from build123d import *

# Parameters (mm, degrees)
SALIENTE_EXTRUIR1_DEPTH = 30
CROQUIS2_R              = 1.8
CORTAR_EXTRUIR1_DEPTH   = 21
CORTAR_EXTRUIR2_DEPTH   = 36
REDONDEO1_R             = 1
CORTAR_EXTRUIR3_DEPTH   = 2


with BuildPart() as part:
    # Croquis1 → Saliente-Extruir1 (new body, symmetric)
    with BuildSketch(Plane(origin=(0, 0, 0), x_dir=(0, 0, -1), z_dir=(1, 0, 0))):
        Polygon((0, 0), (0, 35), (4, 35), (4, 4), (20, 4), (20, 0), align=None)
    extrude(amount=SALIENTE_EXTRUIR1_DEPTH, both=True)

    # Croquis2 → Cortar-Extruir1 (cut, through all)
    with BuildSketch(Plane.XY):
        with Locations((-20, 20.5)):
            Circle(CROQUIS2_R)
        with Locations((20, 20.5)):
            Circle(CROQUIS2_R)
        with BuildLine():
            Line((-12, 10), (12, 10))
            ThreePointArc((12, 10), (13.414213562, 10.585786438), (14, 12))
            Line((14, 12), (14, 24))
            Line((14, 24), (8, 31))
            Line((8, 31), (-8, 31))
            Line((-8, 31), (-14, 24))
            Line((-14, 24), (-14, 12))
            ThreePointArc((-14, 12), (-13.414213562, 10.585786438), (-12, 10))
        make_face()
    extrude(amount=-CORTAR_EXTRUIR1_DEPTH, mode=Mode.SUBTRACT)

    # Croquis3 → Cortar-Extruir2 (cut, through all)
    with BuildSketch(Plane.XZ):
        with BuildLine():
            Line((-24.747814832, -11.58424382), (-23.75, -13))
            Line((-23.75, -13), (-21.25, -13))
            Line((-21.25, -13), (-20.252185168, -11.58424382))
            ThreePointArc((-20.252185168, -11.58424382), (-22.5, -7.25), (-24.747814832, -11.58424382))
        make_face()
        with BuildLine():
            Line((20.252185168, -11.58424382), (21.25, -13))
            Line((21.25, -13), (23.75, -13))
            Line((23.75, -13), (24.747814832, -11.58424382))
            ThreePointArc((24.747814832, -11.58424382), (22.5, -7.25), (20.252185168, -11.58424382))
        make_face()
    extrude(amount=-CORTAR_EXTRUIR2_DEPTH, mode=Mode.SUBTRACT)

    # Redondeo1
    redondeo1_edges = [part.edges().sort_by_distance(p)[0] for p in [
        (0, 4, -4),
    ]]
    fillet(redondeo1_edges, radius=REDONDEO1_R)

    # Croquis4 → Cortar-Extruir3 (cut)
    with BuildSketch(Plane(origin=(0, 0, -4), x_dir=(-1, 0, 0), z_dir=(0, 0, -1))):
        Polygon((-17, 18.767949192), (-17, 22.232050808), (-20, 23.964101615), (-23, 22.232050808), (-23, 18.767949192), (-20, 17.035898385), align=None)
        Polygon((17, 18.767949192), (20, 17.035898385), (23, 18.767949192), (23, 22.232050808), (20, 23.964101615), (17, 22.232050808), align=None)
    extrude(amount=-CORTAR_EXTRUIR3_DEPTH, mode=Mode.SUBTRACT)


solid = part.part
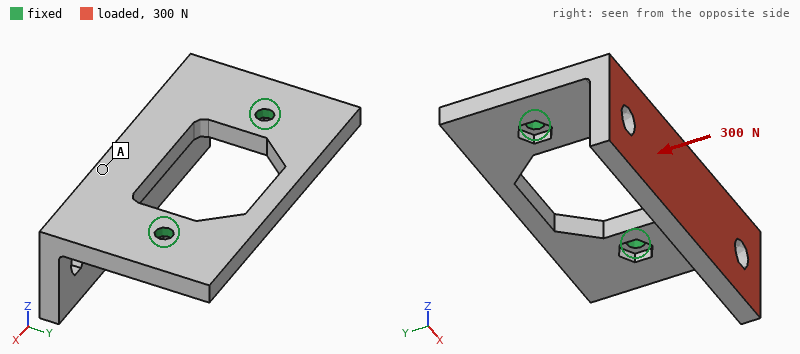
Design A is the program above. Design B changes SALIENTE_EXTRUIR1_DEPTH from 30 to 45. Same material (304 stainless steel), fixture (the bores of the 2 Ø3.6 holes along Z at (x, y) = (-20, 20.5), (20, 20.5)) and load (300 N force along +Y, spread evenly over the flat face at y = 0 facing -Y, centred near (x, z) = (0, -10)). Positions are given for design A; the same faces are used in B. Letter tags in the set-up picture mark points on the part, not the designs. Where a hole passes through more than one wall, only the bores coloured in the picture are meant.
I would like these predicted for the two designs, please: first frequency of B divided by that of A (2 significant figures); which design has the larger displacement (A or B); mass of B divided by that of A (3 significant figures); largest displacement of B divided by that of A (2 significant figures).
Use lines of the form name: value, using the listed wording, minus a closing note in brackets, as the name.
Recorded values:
first frequency of B divided by that of A: 0.88
which design has the larger displacement: A
mass of B divided by that of A: 1.63
largest displacement of B divided by that of A: 0.75
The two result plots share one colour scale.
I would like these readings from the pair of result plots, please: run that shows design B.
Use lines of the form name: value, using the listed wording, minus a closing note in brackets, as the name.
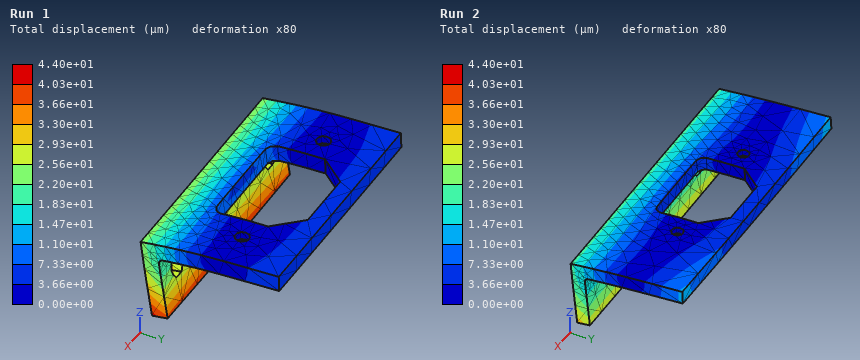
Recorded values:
run that shows design B: Run 2
